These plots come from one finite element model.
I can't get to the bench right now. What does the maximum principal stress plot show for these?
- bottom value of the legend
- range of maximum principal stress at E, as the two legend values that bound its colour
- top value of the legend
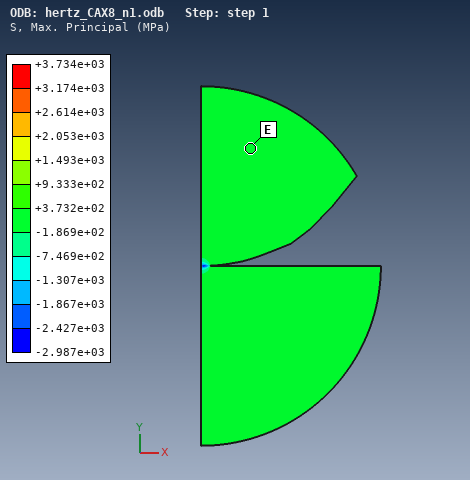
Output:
-2.987e+03 MPa
-1.869e+02 to +3.732e+02 MPa
+3.734e+03 MPa
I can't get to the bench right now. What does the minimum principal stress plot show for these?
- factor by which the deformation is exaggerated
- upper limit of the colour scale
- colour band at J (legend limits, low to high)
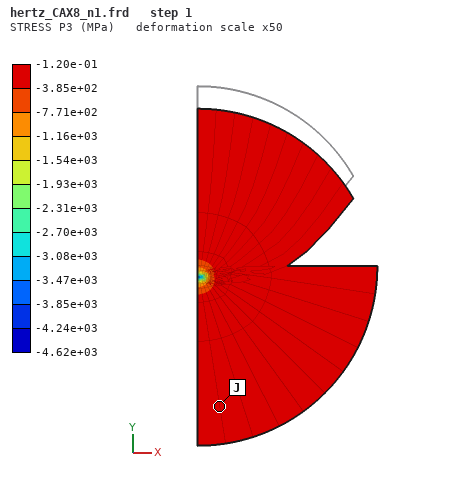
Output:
50
-1.20e-01 MPa
-3.85e+02 to -1.20e-01 MPa
